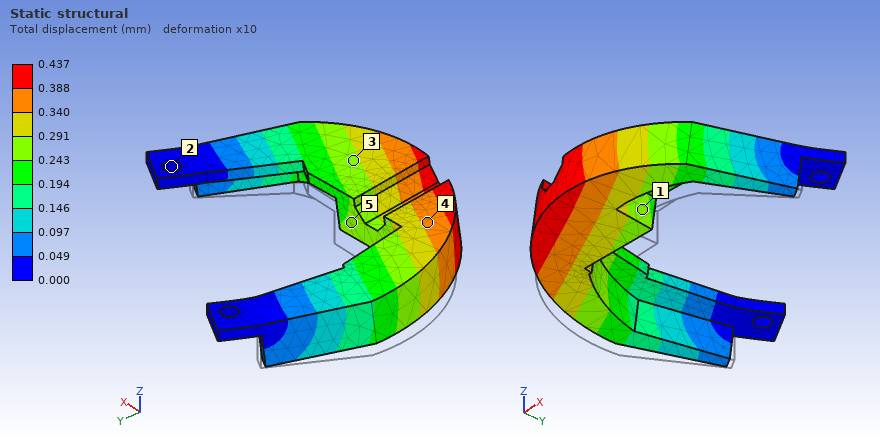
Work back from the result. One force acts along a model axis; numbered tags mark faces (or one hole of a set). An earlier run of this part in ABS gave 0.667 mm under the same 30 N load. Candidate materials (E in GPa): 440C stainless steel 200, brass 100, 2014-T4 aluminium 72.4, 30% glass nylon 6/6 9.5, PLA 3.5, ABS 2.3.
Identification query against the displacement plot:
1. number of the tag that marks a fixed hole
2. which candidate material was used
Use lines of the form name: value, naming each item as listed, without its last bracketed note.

number of the tag that marks a fixed hole: 2
which candidate material was used: PLA
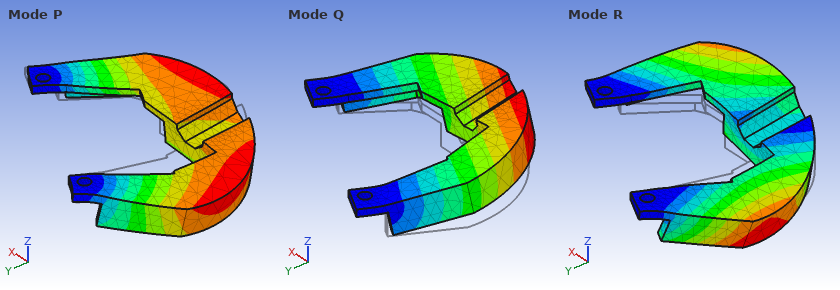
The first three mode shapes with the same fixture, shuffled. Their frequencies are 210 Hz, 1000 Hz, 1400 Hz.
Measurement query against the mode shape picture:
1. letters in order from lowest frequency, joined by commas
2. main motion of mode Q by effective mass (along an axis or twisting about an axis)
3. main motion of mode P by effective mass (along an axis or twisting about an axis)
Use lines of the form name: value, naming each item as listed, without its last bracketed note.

letters in order from lowest frequency, joined by commas: Q, R, P
main motion of mode Q by effective mass: along Z
main motion of mode P by effective mass: along X
